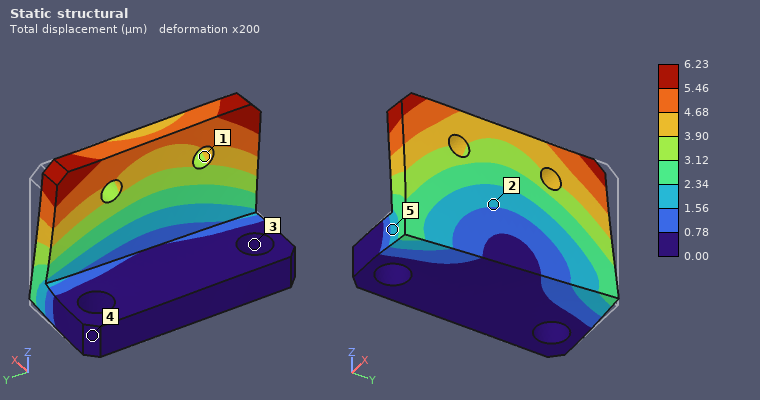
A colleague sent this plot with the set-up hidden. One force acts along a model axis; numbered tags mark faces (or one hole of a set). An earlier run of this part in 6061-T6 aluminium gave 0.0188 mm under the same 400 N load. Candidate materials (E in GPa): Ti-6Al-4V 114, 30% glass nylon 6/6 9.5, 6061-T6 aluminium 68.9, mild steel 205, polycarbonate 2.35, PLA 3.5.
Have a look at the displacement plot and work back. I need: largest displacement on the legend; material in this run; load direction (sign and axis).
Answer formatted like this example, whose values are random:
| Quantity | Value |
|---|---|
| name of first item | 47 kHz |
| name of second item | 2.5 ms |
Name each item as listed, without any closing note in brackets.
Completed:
| Quantity | Value |
|---|---|
| largest displacement on the legend | 6.23 µm |
| material in this run | mild steel |
| load direction | -Y |
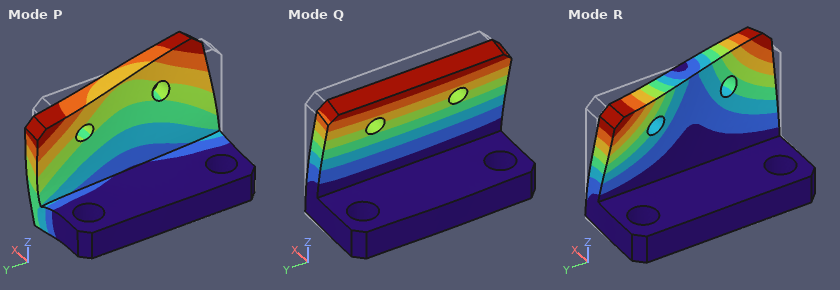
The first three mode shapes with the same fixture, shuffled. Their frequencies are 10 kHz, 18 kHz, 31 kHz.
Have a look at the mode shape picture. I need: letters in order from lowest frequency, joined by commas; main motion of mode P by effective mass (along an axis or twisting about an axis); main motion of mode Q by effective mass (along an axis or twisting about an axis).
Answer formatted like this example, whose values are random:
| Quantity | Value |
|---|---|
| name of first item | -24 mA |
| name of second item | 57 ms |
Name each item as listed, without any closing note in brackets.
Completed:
| Quantity | Value |
|---|---|
| letters in order from lowest frequency, joined by commas | Q, R, P |
| main motion of mode P by effective mass | along Y |
| main motion of mode Q by effective mass | along X |
